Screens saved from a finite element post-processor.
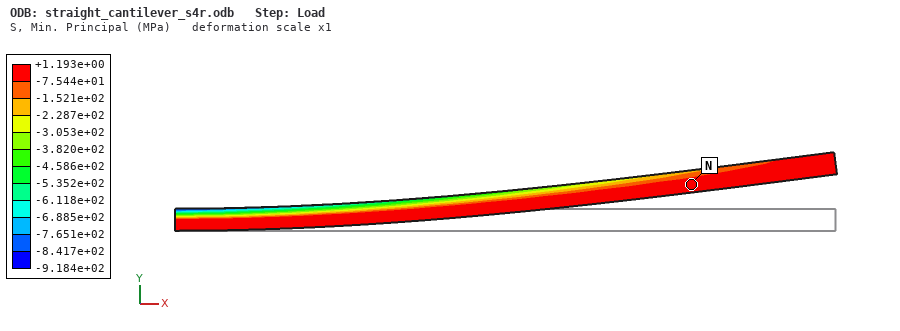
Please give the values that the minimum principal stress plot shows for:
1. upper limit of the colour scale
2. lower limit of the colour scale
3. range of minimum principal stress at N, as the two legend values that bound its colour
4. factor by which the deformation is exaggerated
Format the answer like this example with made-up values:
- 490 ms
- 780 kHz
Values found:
- +1.193e+00 MPa
- -9.184e+02 MPa
- -7.544e+01 to +1.193e+00 MPa
- 1
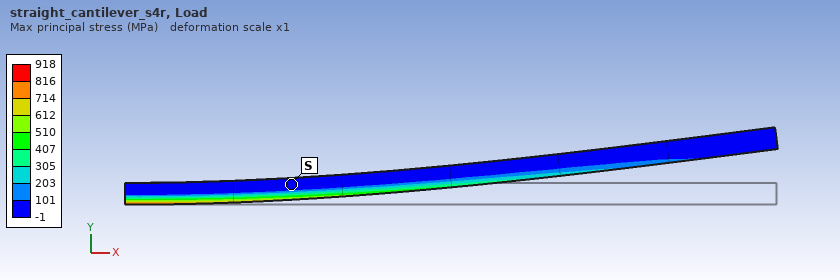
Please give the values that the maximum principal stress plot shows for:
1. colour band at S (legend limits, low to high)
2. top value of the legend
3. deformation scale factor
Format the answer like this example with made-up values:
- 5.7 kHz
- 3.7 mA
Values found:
- -1 to 101 MPa
- 918 MPa
- 1
